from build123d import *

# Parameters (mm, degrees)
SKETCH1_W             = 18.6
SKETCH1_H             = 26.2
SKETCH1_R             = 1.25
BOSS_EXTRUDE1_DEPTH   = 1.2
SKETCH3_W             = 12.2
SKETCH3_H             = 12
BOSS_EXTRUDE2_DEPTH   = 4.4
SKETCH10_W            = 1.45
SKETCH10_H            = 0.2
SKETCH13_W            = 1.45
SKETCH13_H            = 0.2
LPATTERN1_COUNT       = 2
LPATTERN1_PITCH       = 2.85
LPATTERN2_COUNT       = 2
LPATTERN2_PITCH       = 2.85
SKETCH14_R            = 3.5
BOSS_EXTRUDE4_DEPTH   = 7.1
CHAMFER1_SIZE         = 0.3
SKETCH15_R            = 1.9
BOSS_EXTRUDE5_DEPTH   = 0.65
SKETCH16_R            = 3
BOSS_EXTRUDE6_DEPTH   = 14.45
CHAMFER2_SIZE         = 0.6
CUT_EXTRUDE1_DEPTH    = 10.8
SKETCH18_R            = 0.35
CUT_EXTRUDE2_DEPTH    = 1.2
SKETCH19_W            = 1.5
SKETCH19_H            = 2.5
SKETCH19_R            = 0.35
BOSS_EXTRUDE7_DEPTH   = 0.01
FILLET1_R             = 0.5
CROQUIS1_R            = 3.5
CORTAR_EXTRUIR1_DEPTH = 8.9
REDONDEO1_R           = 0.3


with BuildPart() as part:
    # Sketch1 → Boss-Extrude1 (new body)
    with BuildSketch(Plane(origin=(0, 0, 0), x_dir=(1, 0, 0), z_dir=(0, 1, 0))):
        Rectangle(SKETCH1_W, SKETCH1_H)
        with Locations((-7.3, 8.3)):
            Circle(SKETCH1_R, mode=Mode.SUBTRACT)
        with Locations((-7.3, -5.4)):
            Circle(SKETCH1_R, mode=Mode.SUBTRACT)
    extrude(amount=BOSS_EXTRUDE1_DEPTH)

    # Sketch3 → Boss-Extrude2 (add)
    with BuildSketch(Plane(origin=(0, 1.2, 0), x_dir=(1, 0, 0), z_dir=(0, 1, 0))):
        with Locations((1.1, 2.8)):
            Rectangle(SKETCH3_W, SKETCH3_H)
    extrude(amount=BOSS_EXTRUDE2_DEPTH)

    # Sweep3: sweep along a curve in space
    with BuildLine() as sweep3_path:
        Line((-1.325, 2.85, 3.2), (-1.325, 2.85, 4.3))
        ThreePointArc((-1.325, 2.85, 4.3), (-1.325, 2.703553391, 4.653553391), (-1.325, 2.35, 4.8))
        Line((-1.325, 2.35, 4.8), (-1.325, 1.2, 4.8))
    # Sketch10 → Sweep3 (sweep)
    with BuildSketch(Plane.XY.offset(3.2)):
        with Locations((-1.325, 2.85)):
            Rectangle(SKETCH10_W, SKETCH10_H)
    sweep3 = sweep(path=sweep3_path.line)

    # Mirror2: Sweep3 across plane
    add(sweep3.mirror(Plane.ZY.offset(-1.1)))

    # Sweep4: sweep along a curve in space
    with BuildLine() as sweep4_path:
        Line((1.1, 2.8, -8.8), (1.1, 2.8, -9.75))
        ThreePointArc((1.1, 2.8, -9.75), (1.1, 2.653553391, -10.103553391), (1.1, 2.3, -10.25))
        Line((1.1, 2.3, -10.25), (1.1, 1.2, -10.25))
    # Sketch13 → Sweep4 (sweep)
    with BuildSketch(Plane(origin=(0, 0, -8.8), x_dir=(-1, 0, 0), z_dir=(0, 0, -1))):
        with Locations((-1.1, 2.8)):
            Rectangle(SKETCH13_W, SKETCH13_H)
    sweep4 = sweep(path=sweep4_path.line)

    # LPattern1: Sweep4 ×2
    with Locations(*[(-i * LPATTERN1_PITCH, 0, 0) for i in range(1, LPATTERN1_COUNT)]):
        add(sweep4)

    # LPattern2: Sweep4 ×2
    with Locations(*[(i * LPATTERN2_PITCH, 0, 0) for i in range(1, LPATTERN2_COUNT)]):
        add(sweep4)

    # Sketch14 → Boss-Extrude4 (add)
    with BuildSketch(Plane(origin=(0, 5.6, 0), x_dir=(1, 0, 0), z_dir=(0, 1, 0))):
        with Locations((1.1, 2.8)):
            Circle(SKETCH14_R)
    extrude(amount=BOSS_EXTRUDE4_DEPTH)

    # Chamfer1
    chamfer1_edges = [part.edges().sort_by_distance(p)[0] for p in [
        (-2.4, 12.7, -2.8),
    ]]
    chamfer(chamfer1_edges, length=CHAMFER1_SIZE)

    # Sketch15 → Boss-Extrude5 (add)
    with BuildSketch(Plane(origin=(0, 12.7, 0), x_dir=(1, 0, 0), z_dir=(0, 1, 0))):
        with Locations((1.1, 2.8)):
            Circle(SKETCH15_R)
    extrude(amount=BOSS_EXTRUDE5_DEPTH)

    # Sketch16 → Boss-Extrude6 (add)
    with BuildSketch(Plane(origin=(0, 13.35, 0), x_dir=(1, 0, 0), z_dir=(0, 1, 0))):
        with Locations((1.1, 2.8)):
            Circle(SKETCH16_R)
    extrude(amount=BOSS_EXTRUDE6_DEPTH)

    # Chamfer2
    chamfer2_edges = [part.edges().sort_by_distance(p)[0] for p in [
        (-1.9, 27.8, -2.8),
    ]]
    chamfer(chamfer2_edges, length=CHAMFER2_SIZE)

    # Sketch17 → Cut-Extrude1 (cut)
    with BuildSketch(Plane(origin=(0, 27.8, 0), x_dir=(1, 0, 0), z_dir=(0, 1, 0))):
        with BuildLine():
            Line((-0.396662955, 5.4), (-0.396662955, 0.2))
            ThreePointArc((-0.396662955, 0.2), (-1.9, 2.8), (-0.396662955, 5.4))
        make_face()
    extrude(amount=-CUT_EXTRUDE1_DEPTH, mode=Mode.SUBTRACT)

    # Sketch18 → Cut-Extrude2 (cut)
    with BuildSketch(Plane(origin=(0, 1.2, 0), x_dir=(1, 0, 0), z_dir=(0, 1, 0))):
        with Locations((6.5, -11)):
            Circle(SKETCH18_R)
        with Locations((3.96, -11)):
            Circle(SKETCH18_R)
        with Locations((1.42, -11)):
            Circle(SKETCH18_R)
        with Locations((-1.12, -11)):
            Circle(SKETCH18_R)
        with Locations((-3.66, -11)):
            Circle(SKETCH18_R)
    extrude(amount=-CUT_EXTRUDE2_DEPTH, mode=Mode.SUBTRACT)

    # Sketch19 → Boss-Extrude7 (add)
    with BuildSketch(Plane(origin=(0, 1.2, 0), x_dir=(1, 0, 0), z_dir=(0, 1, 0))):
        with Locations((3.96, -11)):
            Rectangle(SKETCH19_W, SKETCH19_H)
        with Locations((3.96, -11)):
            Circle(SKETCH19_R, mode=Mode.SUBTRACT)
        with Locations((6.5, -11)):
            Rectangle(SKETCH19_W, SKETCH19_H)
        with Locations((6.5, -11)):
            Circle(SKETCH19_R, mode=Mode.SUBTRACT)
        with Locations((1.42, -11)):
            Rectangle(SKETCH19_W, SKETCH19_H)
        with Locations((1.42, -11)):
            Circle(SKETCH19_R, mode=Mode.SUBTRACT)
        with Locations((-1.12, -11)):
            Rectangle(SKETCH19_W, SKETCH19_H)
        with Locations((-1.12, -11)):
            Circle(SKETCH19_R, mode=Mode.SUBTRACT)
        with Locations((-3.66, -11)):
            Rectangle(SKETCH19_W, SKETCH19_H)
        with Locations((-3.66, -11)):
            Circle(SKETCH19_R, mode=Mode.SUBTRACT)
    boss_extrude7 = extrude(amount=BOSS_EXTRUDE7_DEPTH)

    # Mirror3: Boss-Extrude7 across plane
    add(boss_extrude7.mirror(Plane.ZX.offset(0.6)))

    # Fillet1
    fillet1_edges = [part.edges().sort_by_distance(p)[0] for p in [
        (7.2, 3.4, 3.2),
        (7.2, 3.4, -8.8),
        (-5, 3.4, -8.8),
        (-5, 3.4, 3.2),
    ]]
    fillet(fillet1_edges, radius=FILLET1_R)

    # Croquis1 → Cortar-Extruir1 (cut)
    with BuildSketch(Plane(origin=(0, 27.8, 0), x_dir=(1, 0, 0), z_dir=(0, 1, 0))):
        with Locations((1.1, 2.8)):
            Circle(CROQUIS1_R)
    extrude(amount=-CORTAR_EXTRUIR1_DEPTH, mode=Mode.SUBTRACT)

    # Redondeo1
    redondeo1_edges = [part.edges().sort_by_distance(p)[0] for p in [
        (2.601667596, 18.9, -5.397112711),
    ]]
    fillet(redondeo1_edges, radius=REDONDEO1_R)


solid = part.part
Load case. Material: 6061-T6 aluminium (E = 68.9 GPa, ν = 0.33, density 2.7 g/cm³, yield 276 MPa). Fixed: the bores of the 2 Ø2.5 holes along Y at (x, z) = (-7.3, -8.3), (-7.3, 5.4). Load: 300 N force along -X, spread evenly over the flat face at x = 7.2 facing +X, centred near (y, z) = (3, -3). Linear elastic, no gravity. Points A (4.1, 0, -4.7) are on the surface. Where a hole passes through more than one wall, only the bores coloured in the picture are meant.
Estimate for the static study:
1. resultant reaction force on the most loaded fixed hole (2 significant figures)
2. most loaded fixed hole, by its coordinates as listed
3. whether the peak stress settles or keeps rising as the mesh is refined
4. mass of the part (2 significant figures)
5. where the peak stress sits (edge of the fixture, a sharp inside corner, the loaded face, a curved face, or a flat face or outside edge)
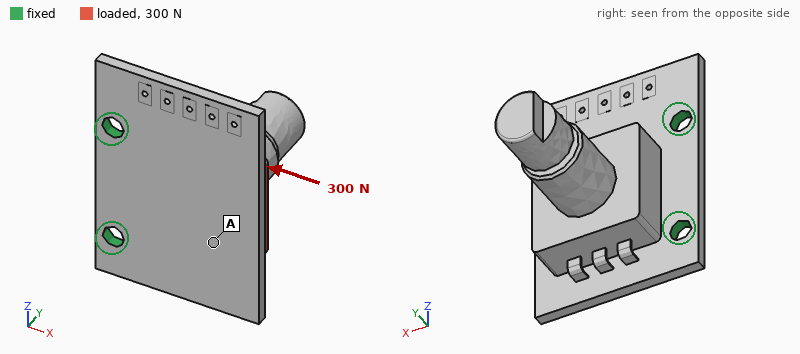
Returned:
180 N
(-7.3, -8.3)
keeps rising
4.4 g
edge of the fixture
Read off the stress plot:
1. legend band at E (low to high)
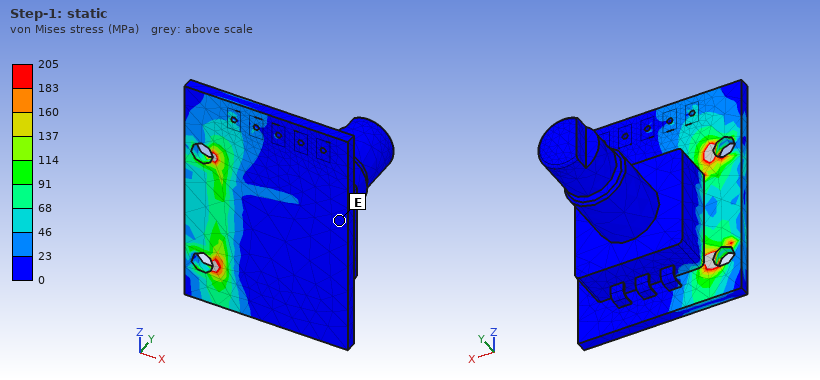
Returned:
0 to 23 MPa
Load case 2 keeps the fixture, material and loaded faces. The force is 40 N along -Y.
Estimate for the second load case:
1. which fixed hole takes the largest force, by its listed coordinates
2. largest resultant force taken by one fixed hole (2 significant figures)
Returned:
(-7.3, -8.3)
22 N
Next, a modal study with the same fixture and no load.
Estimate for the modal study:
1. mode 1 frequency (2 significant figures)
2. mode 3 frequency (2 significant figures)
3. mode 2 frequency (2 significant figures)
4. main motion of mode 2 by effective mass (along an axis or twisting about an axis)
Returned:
2200 Hz
12 kHz
8700 Hz
along Z
